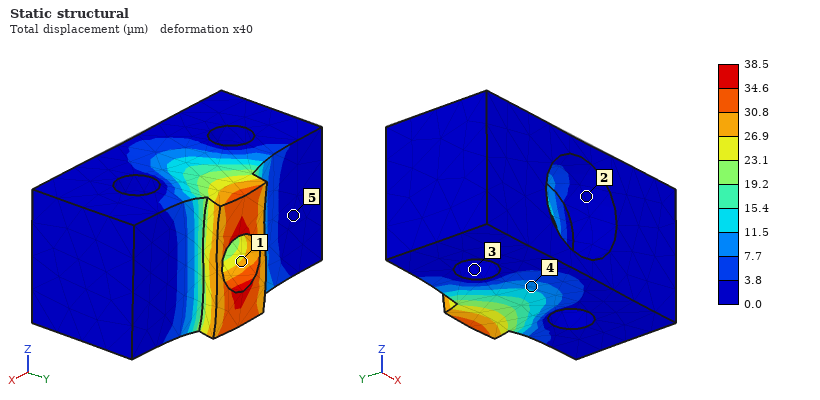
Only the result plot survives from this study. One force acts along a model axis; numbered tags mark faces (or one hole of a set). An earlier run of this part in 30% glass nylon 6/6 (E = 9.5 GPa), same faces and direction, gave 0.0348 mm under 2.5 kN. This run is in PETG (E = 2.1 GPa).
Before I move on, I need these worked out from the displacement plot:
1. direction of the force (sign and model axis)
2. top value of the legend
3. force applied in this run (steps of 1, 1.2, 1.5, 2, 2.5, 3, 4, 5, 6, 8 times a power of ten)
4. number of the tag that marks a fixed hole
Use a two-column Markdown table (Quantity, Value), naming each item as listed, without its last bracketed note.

| Quantity | Value |
|---|---|
| direction of the force | -Z |
| top value of the legend | 38.5 µm |
| force applied in this run | 600 N |
| number of the tag that marks a fixed hole | 3 |
